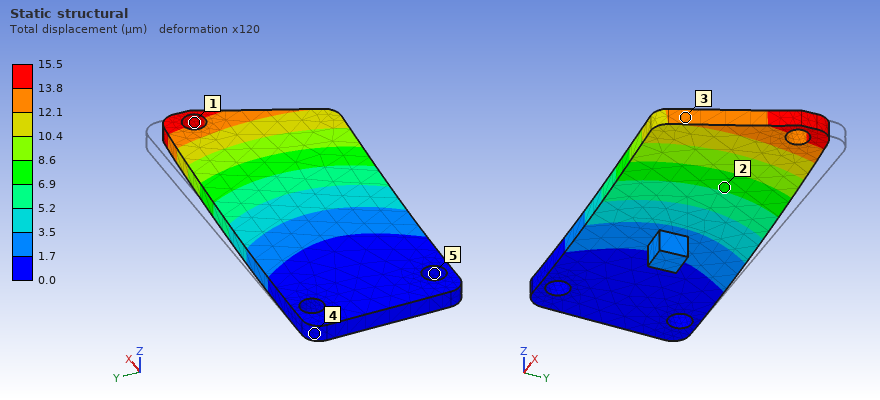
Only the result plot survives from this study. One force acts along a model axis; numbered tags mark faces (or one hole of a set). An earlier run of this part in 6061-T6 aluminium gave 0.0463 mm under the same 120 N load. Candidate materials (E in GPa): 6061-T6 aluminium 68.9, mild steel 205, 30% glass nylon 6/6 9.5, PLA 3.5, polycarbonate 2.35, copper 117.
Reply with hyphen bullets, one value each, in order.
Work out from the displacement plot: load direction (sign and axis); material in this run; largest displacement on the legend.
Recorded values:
- -Y
- mild steel
- 15.5 µm
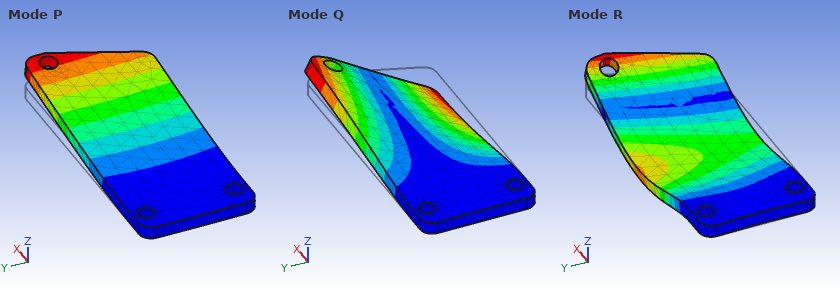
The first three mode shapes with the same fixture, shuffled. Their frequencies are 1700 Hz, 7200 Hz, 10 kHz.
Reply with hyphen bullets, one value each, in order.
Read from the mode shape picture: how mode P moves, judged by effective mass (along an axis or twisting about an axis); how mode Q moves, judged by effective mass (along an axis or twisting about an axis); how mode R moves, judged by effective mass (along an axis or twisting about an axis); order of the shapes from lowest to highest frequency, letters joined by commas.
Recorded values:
- along Z
- twisting about X
- along Z
- P, Q, R
